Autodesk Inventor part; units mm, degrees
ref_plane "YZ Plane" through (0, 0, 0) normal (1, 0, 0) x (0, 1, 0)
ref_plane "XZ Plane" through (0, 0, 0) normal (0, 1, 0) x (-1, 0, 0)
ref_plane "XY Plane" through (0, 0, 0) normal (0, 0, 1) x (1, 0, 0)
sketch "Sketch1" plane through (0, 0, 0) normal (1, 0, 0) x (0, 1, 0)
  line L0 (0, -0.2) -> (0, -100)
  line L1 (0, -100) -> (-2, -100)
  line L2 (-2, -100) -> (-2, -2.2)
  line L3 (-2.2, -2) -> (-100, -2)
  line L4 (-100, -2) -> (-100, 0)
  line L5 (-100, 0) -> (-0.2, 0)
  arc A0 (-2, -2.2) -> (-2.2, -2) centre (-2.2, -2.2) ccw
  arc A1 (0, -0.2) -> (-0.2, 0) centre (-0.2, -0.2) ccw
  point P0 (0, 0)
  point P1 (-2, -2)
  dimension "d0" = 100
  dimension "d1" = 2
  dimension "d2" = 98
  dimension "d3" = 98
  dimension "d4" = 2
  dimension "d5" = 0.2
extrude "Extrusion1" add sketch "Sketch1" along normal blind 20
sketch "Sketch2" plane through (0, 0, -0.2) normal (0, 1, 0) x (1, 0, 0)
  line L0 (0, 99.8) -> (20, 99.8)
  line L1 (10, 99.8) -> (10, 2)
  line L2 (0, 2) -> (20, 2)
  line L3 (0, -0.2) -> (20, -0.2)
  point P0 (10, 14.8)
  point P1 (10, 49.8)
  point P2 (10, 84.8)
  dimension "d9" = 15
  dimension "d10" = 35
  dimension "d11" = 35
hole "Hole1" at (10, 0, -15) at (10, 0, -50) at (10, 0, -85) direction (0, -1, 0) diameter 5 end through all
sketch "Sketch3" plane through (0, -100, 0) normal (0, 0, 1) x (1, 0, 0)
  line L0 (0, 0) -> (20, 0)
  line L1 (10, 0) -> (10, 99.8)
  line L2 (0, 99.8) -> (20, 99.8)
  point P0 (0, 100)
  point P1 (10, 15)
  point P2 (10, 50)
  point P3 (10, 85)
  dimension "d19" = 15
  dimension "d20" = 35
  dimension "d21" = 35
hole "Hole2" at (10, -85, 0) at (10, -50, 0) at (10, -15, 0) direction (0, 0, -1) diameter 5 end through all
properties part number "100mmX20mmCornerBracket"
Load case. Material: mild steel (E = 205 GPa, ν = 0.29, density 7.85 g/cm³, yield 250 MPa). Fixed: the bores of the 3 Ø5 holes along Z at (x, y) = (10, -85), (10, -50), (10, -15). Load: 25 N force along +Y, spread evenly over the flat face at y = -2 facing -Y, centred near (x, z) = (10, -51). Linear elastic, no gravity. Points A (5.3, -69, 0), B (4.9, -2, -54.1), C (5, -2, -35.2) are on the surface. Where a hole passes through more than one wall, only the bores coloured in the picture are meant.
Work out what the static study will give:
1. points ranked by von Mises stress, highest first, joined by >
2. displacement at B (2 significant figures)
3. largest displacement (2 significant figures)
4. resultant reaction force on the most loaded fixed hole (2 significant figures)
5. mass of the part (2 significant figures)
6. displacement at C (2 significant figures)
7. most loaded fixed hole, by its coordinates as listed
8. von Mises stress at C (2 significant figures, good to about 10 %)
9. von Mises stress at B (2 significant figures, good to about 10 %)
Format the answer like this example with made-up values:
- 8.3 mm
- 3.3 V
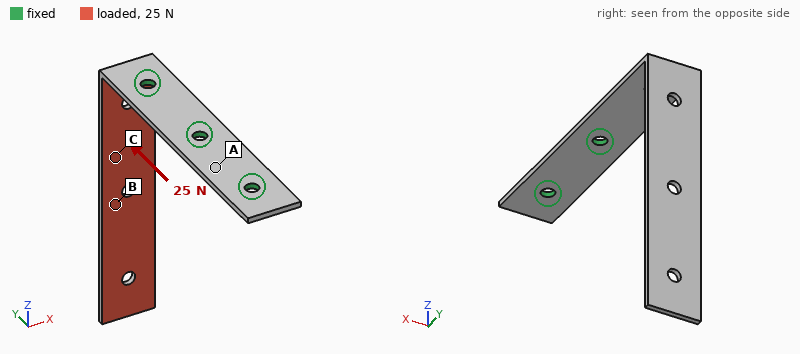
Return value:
- C > B > A
- 0.75 mm
- 1.7 mm
- 24 N
- 60 g
- 0.40 mm
- (10, -15)
- 40 MPa
- 22 MPa
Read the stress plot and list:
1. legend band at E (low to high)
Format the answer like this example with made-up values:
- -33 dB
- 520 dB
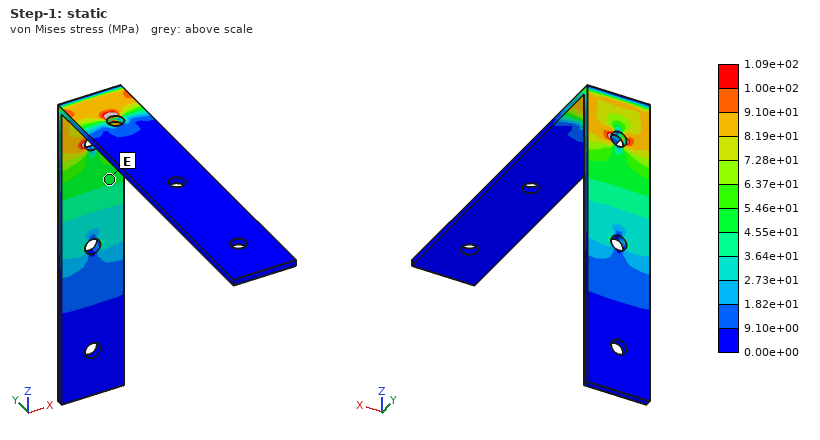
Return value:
- 4.55e+01 to 5.46e+01 MPa
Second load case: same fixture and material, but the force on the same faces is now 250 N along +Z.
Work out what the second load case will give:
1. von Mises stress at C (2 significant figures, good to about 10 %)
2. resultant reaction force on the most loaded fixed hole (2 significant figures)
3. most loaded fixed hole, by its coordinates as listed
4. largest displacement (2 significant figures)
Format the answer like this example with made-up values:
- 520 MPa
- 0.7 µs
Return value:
- 16 MPa
- 250 N
- (10, -15)
- 0.31 mm
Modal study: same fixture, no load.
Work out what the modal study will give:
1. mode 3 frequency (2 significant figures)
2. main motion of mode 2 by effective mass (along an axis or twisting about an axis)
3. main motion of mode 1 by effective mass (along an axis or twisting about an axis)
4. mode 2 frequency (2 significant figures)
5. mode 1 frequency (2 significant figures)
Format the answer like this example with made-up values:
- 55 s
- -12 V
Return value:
- 890 Hz
- along X
- along Y
- 320 Hz
- 140 Hz
